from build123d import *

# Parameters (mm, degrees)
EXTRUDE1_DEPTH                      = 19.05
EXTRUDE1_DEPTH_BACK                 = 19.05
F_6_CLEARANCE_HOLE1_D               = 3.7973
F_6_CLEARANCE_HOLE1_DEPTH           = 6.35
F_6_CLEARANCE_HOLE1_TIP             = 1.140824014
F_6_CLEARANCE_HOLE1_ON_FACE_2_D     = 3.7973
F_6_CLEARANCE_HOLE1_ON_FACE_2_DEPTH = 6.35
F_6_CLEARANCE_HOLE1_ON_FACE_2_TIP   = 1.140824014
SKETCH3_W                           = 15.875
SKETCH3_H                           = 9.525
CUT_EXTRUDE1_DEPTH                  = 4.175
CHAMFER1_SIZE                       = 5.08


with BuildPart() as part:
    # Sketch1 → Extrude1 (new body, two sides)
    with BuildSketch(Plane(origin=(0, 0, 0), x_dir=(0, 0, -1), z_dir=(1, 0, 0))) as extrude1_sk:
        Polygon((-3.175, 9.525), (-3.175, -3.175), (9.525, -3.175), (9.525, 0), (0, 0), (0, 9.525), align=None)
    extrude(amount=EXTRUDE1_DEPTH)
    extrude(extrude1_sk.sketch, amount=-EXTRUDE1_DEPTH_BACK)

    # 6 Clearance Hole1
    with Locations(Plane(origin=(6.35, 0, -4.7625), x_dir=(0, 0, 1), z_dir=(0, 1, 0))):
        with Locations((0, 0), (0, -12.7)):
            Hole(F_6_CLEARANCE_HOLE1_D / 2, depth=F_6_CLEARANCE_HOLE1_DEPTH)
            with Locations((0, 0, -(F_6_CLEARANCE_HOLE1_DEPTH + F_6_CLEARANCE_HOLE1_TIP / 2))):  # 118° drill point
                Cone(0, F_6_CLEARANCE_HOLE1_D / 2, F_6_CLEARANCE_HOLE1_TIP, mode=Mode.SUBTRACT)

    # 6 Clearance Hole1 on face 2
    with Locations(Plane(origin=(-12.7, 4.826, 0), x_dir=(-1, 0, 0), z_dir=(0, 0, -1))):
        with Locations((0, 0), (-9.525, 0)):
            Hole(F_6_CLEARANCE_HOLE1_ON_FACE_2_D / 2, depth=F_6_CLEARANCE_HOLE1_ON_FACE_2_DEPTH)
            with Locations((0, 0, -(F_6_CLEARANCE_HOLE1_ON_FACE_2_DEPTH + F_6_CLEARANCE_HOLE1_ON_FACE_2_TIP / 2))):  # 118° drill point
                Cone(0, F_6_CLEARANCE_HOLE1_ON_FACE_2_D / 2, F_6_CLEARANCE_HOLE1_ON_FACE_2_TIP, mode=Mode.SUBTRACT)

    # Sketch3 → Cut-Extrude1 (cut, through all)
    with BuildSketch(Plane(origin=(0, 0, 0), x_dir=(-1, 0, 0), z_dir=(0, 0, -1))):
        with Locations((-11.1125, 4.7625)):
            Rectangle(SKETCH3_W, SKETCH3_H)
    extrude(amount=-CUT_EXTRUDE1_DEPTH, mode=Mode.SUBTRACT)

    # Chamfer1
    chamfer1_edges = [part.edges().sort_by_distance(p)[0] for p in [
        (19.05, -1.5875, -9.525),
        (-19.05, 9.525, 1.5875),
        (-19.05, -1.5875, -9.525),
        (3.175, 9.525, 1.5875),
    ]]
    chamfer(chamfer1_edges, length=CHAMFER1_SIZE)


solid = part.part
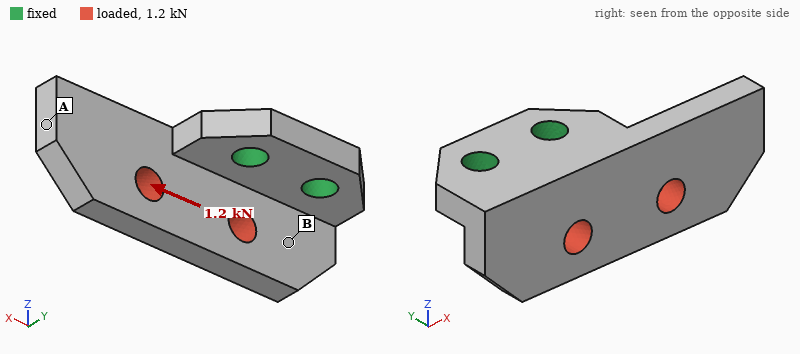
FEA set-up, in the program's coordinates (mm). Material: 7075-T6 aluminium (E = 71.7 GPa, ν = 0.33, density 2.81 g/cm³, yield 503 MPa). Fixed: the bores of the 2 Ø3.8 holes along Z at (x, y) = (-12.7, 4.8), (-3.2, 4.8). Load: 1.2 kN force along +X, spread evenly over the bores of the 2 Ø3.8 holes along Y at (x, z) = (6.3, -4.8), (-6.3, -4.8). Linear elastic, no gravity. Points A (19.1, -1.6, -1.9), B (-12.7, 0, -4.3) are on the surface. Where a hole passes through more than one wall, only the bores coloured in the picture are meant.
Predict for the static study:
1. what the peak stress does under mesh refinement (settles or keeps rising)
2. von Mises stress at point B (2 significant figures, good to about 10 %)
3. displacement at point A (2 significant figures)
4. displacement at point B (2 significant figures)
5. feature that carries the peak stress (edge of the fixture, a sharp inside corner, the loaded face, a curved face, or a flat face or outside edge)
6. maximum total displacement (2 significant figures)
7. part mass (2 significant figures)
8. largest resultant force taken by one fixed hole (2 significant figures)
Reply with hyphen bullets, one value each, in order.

- keeps rising
- 47 MPa
- 73 µm
- 22 µm
- edge of the fixture
- 79 µm
- 5.3 g
- 970 N
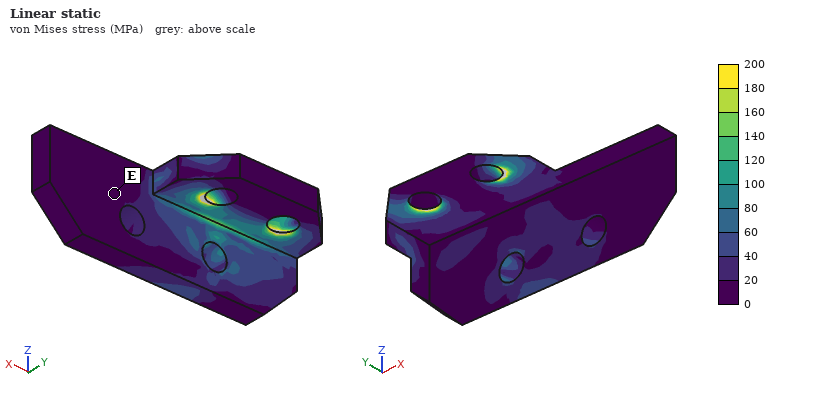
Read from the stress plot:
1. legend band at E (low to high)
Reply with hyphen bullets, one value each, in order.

- 0 to 20 MPa
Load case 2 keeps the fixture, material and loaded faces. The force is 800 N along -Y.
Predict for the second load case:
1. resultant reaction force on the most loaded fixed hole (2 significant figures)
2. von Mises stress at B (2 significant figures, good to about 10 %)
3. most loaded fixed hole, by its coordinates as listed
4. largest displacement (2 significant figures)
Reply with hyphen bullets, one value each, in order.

- 880 N
- 55 MPa
- (-3.2, 4.8)
- 0.22 mm
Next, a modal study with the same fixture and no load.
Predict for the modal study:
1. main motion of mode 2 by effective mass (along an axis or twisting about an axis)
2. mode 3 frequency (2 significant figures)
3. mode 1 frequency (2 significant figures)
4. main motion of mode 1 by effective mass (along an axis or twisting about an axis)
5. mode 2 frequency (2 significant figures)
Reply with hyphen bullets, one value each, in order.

- along Z
- 12 kHz
- 5800 Hz
- along Y
- 8900 Hz
